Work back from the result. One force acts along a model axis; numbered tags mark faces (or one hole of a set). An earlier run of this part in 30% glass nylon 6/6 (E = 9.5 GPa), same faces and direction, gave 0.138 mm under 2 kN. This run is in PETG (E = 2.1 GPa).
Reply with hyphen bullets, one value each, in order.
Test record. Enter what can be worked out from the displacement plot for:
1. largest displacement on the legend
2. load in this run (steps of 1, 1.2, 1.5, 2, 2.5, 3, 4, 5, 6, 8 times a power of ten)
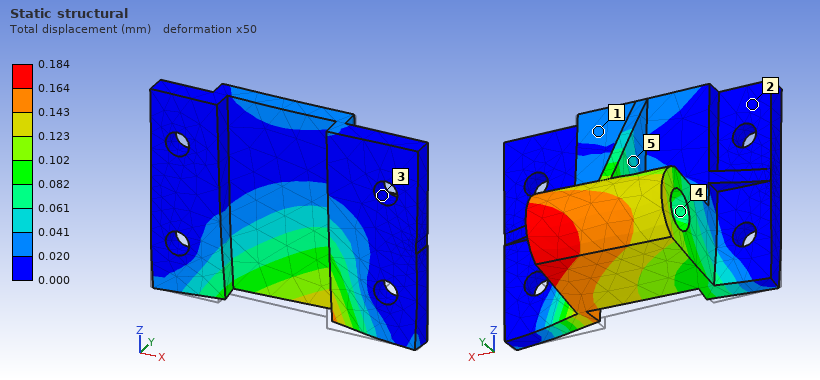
- 0.184 mm
- 600 N
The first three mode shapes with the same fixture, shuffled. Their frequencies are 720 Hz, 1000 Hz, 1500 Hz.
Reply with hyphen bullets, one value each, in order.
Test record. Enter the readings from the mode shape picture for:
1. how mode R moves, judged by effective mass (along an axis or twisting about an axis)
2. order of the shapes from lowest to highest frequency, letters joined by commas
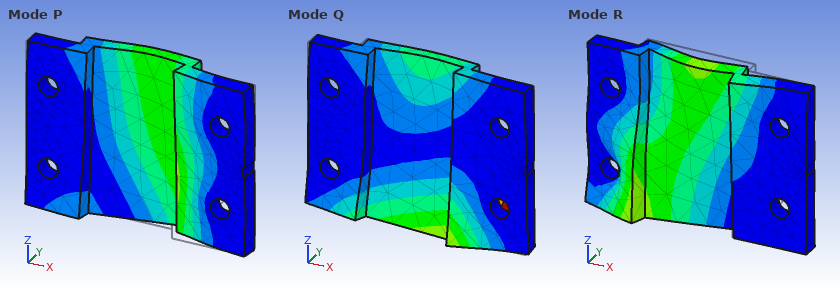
- along Y
- Q, P, R
